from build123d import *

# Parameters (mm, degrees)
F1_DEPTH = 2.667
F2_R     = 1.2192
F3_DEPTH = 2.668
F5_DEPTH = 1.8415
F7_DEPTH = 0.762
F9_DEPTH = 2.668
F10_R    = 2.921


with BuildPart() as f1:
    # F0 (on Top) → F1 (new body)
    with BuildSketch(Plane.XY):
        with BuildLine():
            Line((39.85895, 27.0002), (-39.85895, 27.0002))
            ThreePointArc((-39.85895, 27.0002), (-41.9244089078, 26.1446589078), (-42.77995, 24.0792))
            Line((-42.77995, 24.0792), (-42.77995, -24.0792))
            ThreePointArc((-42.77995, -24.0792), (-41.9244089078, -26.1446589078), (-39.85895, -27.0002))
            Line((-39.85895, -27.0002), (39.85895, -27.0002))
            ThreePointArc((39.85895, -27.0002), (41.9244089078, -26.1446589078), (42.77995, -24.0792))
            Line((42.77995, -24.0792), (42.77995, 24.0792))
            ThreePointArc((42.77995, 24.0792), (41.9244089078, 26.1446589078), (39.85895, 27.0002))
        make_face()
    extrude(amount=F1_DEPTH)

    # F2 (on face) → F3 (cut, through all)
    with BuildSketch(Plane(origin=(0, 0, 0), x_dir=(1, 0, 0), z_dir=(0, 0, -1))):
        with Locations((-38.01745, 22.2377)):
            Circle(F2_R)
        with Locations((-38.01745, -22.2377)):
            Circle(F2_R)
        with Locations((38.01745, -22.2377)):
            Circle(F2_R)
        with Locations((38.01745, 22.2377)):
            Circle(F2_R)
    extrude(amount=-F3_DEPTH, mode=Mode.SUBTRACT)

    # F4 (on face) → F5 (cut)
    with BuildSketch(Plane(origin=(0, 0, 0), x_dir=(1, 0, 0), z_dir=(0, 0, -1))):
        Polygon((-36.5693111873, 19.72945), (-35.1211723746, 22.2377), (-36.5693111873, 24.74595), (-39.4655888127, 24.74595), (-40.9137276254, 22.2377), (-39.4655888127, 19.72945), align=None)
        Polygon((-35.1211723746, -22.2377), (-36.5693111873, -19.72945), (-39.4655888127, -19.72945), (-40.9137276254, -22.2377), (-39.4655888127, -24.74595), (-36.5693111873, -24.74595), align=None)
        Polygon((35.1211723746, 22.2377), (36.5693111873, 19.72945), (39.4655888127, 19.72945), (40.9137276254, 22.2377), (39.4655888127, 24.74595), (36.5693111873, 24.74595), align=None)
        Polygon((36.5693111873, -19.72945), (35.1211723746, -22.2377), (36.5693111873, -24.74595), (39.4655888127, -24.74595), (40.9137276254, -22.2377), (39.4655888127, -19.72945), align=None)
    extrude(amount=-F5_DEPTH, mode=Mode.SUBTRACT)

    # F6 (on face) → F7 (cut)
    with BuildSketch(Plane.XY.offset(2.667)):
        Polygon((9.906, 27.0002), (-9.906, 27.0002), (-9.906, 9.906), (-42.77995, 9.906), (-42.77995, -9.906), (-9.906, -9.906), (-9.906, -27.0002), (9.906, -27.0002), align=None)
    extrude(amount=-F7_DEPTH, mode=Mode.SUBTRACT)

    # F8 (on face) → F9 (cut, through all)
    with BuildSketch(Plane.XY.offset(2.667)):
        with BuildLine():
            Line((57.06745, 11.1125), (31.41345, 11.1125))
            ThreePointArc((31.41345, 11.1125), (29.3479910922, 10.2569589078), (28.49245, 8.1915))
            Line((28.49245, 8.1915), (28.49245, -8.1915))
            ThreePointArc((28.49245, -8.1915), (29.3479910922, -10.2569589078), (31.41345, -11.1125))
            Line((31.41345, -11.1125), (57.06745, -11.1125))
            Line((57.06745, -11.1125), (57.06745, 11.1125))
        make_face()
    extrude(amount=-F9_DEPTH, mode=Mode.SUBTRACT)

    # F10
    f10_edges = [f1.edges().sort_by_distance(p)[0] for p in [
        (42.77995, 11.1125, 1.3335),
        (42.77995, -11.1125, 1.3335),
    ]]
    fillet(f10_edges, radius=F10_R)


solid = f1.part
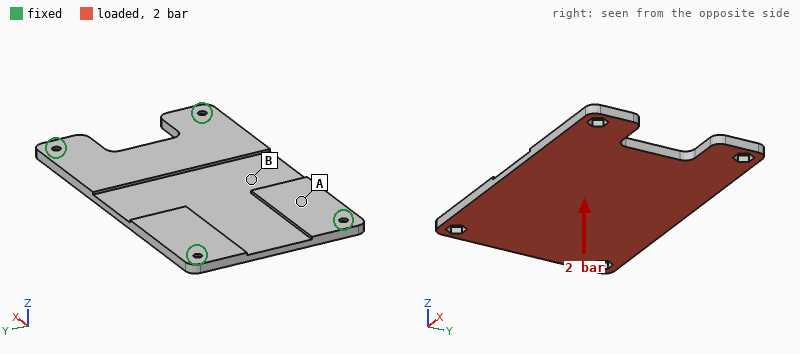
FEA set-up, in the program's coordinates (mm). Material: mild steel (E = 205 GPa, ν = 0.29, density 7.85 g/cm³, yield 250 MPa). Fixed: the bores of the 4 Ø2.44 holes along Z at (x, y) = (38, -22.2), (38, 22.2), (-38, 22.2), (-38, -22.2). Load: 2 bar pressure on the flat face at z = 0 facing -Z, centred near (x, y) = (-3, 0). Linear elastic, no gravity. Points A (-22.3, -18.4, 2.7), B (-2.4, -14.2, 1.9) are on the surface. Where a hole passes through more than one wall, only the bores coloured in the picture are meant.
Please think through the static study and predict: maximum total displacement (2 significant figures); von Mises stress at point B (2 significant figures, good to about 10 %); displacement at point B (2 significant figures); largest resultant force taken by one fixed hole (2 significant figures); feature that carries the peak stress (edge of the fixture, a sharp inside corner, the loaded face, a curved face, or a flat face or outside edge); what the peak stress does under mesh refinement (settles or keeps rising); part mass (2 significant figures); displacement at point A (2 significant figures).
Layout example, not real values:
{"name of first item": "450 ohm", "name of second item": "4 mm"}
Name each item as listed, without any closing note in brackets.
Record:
{"maximum total displacement": "0.17 mm", "von Mises stress at point B": "60 MPa", "displacement at point B": "0.16 mm", "largest resultant force taken by one fixed hole": "1.1 kN", "feature that carries the peak stress": "edge of the fixture", "what the peak stress does under mesh refinement": "keeps rising", "part mass": "78 g", "displacement at point A": "0.083 mm"}
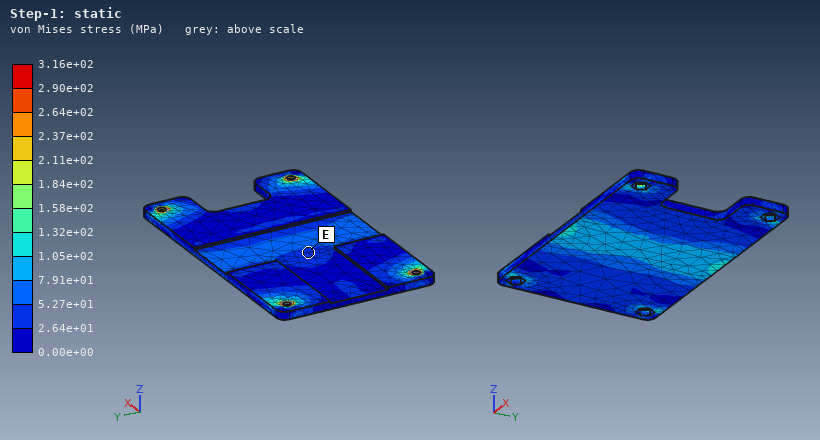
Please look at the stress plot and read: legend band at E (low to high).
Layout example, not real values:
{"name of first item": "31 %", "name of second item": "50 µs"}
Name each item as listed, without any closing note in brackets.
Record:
{"legend band at E": "2.64e+01 to 5.27e+01 MPa"}
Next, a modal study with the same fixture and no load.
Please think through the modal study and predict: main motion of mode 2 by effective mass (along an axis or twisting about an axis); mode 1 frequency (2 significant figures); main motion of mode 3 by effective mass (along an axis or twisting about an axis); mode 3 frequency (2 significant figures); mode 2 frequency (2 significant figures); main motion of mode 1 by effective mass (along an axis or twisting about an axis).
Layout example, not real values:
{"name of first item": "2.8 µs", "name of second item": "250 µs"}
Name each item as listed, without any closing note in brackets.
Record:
{"main motion of mode 2 by effective mass": "twisting about X", "mode 1 frequency": "1500 Hz", "main motion of mode 3 by effective mass": "twisting about Y", "mode 3 frequency": "3900 Hz", "mode 2 frequency": "2600 Hz", "main motion of mode 1 by effective mass": "along Z"}
